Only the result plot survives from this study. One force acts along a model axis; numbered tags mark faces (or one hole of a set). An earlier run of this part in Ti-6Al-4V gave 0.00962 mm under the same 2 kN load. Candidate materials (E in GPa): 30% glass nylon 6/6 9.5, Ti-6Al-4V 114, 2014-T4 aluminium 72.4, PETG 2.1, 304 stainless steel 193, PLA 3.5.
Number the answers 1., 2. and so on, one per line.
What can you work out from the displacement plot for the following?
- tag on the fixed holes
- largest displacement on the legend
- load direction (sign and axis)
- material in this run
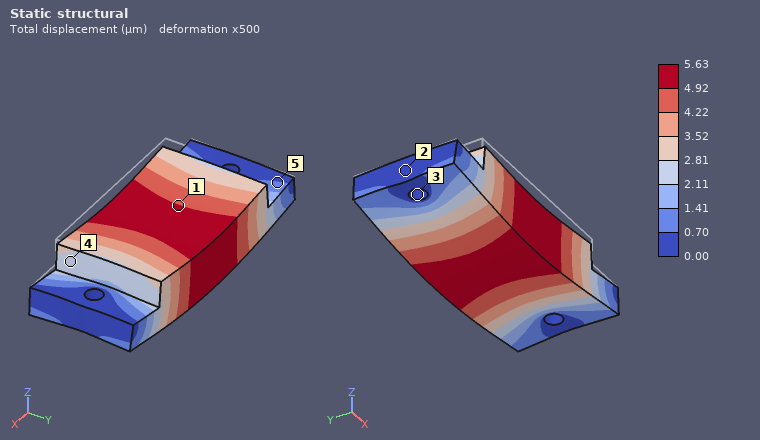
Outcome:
1. 3
2. 5.63 µm
3. -Z
4. 304 stainless steel
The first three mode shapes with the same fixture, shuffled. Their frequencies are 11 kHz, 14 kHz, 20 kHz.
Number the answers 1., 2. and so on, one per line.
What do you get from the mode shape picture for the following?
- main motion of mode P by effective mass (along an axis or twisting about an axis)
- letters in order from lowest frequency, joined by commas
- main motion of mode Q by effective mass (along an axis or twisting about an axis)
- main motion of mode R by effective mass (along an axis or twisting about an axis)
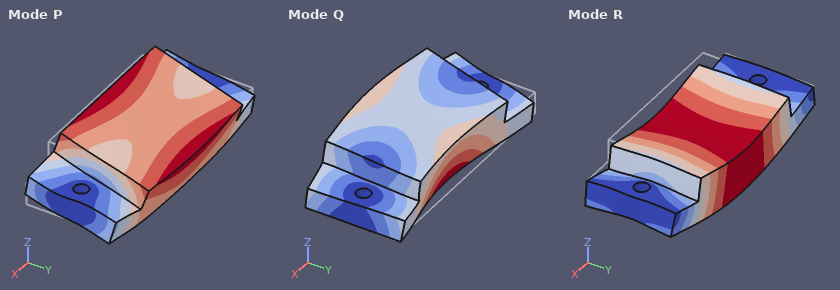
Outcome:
1. along Y
2. P, R, Q
3. along Y
4. along Z
